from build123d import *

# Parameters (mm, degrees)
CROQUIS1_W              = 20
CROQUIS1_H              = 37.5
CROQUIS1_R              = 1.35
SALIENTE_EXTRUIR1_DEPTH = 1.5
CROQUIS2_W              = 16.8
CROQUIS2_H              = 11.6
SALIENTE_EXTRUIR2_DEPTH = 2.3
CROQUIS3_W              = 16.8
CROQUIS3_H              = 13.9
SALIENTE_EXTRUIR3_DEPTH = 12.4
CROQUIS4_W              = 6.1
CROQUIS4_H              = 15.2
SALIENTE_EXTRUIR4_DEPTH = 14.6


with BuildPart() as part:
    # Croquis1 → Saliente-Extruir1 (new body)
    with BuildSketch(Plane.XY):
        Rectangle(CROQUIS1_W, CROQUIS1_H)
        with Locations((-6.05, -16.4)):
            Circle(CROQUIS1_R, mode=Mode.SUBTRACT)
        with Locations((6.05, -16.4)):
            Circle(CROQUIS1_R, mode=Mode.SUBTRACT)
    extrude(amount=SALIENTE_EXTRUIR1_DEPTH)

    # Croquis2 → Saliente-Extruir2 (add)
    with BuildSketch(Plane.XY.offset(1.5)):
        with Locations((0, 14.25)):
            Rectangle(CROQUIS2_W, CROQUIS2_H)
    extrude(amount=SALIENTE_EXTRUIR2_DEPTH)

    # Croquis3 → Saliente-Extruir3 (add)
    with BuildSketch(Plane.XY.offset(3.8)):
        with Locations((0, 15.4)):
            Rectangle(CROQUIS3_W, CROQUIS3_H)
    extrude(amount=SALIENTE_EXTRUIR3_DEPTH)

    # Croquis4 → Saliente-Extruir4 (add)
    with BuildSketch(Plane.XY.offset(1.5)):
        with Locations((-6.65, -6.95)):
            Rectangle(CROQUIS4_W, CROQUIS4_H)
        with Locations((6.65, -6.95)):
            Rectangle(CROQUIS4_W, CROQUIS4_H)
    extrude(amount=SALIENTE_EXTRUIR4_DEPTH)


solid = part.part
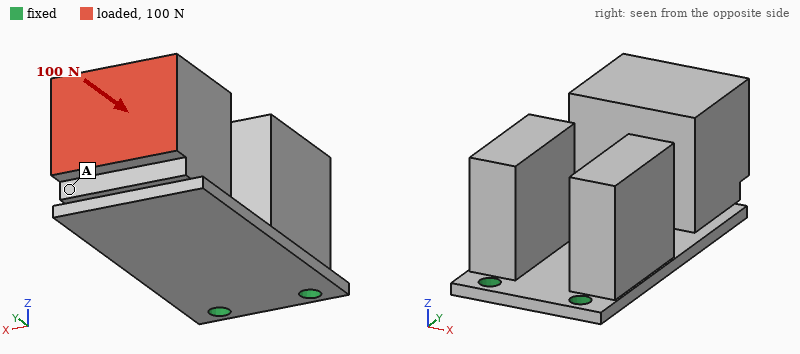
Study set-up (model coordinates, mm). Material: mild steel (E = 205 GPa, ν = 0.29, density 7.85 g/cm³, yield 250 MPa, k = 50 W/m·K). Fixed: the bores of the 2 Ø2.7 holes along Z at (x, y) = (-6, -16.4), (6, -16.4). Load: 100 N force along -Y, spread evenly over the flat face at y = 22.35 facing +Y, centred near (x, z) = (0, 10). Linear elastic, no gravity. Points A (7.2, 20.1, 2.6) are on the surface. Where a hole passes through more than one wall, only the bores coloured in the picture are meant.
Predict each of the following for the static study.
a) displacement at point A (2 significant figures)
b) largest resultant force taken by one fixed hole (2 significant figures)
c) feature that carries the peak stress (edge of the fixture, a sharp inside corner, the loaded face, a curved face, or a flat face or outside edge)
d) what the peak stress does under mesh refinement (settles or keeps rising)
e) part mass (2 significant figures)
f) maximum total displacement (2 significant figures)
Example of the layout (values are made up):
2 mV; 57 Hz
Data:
0.18 mm; 51 N; edge of the fixture; keeps rising; 56 g; 0.24 mm
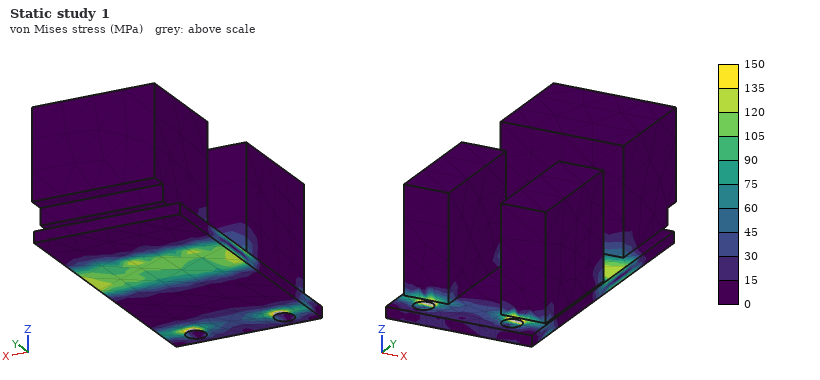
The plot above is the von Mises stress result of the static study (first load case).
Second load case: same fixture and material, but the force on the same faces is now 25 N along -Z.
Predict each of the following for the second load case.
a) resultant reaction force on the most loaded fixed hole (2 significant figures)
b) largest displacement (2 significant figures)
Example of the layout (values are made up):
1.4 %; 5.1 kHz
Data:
17 N; 0.16 mm
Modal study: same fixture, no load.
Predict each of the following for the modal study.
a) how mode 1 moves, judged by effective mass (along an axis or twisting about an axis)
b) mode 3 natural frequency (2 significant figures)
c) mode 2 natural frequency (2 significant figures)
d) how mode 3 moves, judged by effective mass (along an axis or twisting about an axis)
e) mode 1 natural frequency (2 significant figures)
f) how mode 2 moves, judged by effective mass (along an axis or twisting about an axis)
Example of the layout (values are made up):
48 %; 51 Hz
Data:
along Z; 1800 Hz; 1500 Hz; along Z; 490 Hz; along X
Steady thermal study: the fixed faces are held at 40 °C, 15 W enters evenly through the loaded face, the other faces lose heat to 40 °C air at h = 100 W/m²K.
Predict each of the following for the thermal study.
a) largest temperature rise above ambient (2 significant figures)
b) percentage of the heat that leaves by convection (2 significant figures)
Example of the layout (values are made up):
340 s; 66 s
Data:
78 K; 79 %
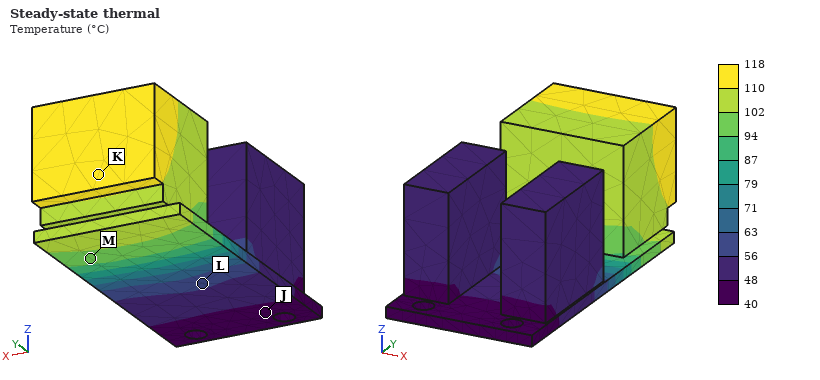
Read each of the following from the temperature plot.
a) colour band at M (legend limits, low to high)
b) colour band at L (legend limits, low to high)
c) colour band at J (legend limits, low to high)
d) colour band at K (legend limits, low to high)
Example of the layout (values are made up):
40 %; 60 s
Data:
94 to 102 °C; 56 to 63 °C; 40 to 48 °C; 110 to 118 °C
